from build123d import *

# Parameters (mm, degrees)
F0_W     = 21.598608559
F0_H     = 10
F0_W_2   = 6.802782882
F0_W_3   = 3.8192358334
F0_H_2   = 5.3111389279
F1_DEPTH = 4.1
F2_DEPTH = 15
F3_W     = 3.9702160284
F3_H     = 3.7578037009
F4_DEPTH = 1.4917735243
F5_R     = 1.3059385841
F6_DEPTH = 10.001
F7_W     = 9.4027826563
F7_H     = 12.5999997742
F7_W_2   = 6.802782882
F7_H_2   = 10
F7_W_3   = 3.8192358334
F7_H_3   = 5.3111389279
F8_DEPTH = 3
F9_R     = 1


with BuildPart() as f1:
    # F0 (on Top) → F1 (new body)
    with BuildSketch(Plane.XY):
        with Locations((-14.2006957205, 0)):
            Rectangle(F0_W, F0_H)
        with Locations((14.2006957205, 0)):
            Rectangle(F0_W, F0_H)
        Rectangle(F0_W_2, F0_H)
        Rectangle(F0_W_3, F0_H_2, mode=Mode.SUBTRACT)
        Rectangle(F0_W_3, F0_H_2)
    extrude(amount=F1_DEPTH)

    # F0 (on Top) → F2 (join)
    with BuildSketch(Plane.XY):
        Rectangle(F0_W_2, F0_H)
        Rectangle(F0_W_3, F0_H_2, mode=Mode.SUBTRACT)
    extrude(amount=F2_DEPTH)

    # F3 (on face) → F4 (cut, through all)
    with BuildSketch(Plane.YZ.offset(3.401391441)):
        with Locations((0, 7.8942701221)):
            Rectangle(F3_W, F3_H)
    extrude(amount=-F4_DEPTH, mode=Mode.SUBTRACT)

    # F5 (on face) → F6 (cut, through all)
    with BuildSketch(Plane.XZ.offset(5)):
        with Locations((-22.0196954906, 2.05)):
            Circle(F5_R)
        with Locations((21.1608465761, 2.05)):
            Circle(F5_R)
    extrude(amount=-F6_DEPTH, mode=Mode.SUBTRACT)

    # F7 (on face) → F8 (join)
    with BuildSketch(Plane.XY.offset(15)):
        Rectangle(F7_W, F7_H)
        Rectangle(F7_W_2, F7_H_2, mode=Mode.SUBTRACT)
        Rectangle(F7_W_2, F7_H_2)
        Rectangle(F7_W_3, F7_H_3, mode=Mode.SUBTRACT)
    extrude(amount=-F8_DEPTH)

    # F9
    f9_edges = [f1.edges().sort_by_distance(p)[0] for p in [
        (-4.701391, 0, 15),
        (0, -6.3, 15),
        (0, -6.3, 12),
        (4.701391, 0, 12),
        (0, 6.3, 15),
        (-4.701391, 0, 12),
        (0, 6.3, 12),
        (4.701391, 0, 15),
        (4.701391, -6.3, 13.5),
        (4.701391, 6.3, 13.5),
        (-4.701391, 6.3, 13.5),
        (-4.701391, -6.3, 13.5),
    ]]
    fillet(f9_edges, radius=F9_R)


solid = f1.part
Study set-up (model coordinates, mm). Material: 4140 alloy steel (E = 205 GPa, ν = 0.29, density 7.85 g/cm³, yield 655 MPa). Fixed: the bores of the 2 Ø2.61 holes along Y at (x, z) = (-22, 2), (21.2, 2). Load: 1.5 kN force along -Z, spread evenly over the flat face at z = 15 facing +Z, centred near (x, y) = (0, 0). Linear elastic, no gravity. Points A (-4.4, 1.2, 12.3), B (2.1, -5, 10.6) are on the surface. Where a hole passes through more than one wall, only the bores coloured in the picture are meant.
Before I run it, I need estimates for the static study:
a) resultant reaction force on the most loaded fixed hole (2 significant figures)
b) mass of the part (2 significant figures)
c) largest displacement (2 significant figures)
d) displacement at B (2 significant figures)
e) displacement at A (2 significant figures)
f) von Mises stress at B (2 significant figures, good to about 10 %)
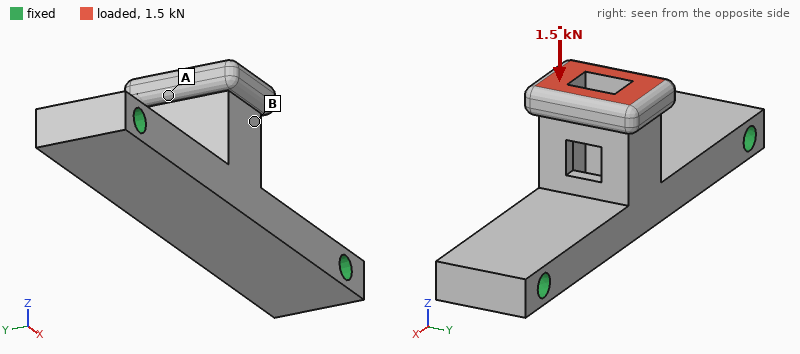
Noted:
790 N
20 g
47 µm
46 µm
47 µm
42 MPa
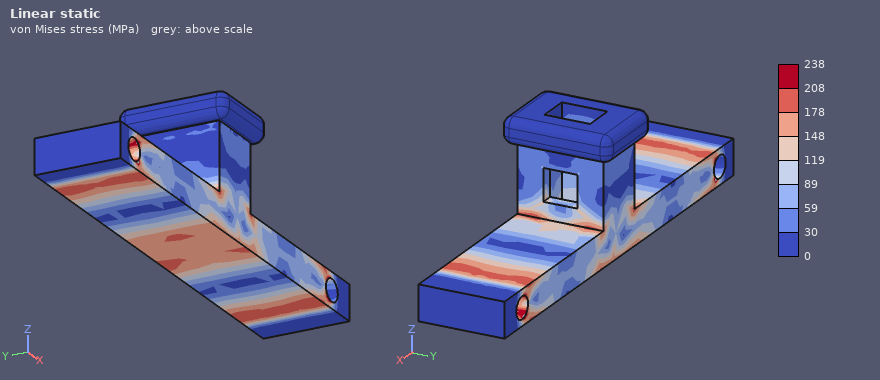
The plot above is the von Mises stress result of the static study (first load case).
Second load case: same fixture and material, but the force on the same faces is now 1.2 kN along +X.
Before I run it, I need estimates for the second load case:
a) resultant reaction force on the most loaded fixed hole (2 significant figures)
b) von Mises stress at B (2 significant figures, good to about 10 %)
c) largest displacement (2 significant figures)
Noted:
820 N
97 MPa
61 µm
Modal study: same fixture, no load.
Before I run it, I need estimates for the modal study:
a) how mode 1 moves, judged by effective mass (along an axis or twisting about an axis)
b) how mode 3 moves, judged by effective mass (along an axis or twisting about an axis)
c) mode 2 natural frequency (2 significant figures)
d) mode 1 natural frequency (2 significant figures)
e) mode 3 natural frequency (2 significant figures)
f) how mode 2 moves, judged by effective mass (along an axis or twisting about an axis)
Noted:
along Y
along X
8800 Hz
8300 Hz
14 kHz
along Z
